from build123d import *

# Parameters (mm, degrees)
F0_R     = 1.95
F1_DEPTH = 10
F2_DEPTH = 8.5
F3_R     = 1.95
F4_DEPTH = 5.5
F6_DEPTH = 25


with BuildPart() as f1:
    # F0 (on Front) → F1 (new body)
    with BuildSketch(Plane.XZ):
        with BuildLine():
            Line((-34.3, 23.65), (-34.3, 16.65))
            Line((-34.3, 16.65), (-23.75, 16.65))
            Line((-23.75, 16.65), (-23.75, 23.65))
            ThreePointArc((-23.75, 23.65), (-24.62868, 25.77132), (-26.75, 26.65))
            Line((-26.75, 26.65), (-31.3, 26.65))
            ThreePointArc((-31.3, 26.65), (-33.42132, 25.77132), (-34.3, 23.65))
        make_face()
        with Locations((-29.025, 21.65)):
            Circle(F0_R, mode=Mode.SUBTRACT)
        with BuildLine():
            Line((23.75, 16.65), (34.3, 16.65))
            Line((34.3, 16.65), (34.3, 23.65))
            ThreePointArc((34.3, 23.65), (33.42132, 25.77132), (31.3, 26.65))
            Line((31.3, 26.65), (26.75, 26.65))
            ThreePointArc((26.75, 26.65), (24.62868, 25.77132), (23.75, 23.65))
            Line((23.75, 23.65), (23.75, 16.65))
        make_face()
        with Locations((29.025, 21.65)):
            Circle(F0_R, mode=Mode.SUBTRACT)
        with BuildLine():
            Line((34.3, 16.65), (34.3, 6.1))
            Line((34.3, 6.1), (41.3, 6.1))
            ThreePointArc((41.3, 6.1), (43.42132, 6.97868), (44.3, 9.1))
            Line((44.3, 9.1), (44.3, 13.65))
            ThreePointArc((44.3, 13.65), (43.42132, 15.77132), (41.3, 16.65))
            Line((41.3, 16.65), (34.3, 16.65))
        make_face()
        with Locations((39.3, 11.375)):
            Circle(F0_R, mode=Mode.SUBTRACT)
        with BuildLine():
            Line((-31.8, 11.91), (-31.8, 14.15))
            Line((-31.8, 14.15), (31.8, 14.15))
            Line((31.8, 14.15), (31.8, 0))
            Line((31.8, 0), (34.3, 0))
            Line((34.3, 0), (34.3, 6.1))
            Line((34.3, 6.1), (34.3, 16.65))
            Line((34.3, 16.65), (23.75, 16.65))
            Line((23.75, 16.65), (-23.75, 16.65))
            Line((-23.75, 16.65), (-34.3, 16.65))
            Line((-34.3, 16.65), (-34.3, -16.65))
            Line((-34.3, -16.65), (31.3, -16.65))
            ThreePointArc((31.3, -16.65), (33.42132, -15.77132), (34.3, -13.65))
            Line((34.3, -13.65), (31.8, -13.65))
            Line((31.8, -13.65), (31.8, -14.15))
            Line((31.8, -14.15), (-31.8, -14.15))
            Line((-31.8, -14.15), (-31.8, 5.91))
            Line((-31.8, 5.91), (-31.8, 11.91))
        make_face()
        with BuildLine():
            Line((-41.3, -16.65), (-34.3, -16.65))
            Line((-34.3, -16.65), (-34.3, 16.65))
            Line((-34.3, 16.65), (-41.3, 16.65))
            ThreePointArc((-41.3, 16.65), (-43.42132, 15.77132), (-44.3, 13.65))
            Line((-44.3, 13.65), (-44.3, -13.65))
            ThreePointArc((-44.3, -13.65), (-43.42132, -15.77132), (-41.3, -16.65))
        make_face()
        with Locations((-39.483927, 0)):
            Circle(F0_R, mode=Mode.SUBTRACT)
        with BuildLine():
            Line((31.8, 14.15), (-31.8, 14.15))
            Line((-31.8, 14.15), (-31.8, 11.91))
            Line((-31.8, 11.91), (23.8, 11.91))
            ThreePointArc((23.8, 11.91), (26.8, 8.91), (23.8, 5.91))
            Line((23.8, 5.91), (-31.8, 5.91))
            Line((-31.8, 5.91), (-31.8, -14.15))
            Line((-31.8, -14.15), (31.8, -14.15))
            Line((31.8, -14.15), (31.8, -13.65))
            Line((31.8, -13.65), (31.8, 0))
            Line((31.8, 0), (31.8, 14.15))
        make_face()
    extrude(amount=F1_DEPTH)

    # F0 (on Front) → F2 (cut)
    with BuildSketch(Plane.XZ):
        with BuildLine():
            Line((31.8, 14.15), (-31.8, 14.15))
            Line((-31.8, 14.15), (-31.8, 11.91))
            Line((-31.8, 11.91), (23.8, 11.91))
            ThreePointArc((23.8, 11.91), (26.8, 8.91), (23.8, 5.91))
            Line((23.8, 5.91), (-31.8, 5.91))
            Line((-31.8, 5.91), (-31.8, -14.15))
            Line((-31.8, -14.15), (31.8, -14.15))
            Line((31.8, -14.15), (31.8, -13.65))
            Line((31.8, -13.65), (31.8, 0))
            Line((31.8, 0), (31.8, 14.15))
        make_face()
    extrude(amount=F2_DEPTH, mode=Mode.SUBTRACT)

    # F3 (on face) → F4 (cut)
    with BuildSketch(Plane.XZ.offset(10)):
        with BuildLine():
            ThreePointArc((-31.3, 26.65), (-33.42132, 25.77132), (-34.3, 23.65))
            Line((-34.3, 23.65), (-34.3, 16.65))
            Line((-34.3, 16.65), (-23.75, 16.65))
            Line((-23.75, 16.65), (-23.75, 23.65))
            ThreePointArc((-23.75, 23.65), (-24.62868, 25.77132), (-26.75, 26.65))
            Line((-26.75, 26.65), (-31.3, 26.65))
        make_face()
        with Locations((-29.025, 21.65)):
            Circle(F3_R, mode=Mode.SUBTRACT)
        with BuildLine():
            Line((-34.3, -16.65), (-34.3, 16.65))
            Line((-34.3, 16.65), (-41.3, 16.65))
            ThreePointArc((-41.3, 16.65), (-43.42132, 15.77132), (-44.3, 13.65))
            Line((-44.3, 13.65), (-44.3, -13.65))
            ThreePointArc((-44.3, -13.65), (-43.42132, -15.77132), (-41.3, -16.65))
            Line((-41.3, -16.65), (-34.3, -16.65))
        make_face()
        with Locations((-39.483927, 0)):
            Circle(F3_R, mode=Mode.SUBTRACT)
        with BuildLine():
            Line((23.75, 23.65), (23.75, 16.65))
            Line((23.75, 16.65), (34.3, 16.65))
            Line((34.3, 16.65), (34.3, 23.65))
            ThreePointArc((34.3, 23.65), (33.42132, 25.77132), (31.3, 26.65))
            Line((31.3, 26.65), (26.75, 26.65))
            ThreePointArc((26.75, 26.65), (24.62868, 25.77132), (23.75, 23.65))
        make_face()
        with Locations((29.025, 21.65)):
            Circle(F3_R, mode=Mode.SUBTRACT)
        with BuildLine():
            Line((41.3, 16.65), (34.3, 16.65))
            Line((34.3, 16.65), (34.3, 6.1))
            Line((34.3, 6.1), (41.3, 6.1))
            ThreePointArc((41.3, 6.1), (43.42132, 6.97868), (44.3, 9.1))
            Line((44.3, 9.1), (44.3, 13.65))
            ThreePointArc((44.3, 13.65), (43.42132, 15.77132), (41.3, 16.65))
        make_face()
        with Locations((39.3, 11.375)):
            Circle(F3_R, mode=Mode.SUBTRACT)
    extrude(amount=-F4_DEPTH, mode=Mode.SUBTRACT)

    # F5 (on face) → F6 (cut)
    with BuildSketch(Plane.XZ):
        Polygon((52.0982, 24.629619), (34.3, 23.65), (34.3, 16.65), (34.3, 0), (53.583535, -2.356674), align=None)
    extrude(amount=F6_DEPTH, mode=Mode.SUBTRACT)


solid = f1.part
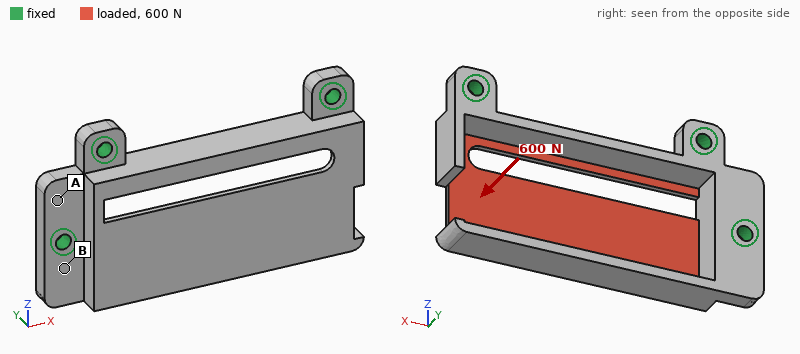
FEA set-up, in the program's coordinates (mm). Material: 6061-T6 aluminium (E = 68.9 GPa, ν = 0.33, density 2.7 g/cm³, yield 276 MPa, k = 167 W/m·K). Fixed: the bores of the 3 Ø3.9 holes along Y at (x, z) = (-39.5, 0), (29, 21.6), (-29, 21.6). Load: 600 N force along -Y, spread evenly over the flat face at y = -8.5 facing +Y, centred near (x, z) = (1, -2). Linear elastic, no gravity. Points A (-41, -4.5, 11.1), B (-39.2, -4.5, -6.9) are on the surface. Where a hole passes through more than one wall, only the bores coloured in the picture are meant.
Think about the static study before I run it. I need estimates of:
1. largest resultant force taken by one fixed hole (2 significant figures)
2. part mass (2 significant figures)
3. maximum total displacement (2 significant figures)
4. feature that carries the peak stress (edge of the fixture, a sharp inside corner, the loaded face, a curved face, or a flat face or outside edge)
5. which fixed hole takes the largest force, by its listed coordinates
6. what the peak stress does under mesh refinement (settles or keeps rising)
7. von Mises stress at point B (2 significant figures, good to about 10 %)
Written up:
580 N
24 g
0.56 mm
a sharp inside corner
(-39.5, 0)
keeps rising
35 MPa
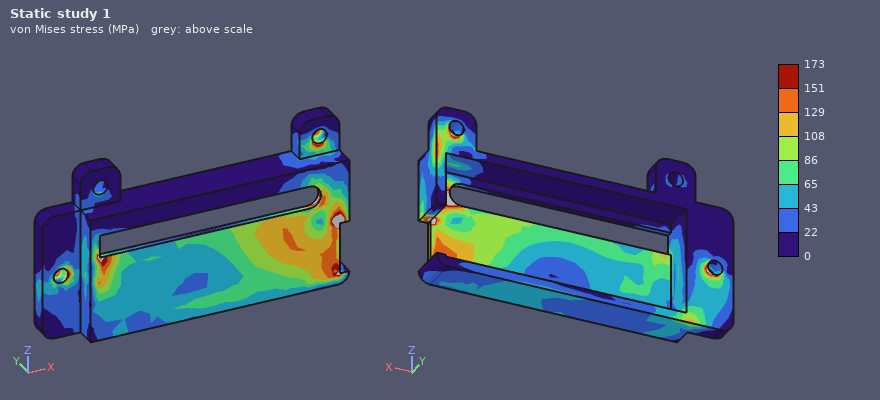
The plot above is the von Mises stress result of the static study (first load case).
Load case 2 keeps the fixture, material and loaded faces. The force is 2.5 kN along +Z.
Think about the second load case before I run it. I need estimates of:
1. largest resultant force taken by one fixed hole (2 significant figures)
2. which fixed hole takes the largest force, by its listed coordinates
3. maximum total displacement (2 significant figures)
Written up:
1.3 kN
(29, 21.6)
0.25 mm
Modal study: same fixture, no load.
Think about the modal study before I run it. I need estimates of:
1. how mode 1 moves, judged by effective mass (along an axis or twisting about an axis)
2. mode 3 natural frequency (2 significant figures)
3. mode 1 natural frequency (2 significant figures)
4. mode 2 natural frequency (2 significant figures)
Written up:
along Y
5000 Hz
1800 Hz
2900 Hz
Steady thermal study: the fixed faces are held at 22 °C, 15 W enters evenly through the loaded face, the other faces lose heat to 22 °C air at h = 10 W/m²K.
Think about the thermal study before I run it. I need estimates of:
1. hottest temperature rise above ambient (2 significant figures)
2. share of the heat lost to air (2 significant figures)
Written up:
30 K
5.7 %
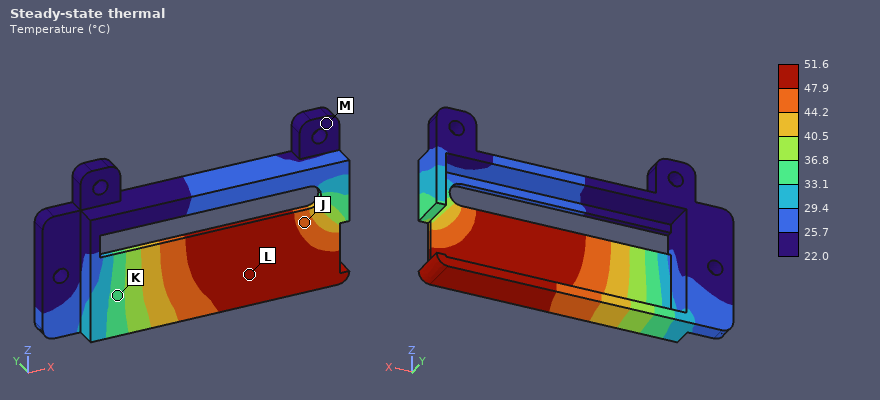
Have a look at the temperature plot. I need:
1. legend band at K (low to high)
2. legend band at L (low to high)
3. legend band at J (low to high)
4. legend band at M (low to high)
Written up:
33.1 to 36.8 °C
47.9 to 51.6 °C
44.2 to 47.9 °C
22.0 to 25.7 °C
